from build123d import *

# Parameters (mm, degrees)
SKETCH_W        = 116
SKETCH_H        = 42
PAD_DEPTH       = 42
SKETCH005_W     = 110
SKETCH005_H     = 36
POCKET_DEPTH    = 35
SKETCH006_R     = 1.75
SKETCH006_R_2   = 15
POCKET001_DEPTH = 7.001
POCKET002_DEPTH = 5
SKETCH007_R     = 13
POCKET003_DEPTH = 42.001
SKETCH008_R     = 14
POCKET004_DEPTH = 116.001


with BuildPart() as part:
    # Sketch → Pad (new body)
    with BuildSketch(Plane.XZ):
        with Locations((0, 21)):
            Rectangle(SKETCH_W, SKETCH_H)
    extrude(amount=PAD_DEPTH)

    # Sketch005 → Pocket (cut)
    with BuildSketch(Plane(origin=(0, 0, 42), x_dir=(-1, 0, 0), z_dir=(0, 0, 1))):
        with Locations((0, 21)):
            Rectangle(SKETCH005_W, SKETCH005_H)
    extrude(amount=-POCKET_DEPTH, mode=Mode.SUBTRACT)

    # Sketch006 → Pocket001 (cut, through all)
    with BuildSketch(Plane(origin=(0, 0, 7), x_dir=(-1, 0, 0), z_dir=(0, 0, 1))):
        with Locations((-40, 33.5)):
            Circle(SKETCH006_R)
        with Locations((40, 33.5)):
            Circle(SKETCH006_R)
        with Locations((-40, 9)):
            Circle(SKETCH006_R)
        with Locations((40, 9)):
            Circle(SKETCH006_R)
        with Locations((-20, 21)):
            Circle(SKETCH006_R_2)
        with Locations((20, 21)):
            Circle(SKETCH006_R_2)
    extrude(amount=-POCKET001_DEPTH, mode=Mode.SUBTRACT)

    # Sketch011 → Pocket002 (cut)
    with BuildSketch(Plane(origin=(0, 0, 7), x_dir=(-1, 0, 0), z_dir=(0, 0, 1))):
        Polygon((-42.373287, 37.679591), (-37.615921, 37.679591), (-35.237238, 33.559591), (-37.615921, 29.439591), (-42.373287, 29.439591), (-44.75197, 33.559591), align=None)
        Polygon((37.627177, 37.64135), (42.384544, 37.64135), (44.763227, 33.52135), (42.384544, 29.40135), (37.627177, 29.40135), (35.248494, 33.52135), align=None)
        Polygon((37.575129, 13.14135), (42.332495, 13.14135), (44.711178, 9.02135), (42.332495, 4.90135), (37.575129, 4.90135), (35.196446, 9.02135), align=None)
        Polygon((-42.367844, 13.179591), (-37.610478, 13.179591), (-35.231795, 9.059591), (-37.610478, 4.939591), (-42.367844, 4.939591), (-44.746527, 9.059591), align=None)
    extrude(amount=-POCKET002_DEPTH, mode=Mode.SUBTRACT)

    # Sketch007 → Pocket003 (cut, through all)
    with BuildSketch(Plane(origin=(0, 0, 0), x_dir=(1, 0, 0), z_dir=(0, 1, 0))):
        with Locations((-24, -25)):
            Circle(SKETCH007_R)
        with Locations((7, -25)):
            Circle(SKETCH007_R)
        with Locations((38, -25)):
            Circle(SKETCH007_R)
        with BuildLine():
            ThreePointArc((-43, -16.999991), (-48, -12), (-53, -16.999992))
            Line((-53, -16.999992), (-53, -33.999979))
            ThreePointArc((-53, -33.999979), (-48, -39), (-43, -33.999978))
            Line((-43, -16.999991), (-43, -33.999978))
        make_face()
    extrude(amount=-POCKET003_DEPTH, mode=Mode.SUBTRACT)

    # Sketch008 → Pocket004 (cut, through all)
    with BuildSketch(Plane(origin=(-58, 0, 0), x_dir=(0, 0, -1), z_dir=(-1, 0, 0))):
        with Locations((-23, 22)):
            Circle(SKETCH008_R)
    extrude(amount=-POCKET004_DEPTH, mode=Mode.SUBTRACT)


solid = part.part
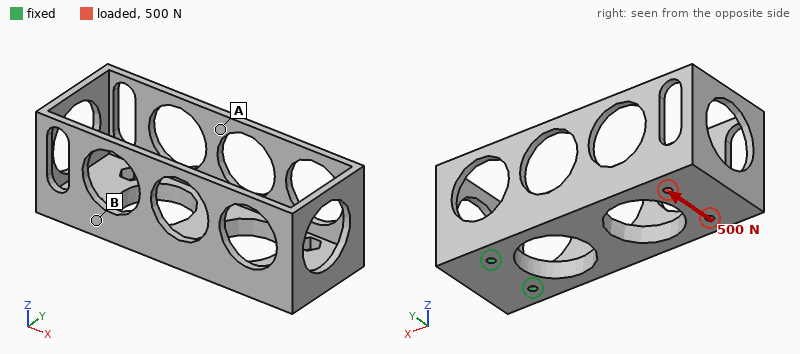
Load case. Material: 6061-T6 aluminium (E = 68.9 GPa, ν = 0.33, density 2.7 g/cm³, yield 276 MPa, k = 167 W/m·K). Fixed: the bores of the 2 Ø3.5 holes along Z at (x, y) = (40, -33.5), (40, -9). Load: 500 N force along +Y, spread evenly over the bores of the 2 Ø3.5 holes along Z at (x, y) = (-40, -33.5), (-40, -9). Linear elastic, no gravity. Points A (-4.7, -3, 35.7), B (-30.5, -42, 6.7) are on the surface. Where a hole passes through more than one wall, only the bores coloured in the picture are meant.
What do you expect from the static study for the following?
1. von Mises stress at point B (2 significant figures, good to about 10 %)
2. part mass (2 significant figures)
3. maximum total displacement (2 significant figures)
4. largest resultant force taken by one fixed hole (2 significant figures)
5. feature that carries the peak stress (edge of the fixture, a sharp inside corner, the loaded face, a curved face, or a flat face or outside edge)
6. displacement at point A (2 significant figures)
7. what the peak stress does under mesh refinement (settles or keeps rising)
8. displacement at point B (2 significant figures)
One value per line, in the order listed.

12 MPa
110 g
0.17 mm
1.5 kN
edge of the fixture
0.058 mm
keeps rising
0.13 mm
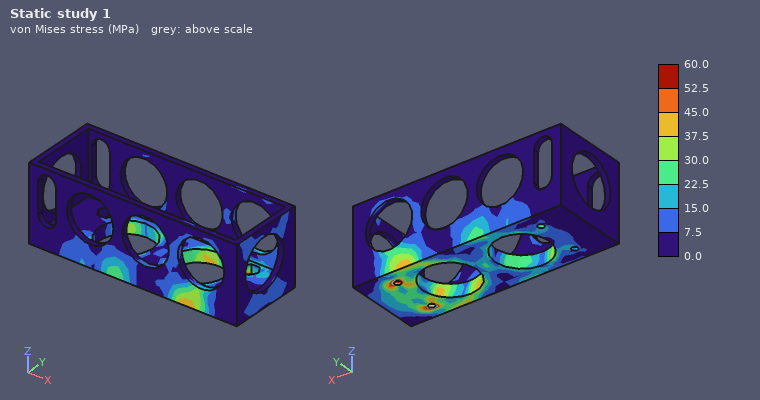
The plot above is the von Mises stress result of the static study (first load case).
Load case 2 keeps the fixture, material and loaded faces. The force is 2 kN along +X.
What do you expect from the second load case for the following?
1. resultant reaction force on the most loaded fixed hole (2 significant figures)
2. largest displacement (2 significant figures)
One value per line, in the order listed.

1.0 kN
80 µm
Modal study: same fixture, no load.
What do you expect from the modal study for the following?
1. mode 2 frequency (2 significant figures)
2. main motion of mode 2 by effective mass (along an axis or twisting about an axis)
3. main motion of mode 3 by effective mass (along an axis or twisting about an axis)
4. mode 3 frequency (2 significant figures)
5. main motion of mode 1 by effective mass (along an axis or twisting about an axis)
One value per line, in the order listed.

970 Hz
along Y
along Y
1500 Hz
along Z
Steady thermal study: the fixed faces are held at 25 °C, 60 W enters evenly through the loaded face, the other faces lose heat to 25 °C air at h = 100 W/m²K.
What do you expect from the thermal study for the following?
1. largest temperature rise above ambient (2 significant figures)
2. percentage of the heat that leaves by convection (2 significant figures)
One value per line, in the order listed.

69 K
85 %
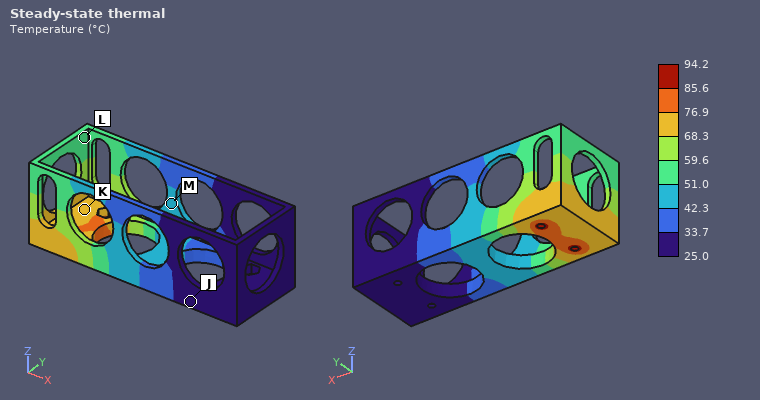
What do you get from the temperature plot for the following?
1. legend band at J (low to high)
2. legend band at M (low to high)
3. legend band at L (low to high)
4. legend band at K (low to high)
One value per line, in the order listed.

25.0 to 33.7 °C
42.3 to 51.0 °C
51.0 to 59.6 °C
68.3 to 76.9 °C
